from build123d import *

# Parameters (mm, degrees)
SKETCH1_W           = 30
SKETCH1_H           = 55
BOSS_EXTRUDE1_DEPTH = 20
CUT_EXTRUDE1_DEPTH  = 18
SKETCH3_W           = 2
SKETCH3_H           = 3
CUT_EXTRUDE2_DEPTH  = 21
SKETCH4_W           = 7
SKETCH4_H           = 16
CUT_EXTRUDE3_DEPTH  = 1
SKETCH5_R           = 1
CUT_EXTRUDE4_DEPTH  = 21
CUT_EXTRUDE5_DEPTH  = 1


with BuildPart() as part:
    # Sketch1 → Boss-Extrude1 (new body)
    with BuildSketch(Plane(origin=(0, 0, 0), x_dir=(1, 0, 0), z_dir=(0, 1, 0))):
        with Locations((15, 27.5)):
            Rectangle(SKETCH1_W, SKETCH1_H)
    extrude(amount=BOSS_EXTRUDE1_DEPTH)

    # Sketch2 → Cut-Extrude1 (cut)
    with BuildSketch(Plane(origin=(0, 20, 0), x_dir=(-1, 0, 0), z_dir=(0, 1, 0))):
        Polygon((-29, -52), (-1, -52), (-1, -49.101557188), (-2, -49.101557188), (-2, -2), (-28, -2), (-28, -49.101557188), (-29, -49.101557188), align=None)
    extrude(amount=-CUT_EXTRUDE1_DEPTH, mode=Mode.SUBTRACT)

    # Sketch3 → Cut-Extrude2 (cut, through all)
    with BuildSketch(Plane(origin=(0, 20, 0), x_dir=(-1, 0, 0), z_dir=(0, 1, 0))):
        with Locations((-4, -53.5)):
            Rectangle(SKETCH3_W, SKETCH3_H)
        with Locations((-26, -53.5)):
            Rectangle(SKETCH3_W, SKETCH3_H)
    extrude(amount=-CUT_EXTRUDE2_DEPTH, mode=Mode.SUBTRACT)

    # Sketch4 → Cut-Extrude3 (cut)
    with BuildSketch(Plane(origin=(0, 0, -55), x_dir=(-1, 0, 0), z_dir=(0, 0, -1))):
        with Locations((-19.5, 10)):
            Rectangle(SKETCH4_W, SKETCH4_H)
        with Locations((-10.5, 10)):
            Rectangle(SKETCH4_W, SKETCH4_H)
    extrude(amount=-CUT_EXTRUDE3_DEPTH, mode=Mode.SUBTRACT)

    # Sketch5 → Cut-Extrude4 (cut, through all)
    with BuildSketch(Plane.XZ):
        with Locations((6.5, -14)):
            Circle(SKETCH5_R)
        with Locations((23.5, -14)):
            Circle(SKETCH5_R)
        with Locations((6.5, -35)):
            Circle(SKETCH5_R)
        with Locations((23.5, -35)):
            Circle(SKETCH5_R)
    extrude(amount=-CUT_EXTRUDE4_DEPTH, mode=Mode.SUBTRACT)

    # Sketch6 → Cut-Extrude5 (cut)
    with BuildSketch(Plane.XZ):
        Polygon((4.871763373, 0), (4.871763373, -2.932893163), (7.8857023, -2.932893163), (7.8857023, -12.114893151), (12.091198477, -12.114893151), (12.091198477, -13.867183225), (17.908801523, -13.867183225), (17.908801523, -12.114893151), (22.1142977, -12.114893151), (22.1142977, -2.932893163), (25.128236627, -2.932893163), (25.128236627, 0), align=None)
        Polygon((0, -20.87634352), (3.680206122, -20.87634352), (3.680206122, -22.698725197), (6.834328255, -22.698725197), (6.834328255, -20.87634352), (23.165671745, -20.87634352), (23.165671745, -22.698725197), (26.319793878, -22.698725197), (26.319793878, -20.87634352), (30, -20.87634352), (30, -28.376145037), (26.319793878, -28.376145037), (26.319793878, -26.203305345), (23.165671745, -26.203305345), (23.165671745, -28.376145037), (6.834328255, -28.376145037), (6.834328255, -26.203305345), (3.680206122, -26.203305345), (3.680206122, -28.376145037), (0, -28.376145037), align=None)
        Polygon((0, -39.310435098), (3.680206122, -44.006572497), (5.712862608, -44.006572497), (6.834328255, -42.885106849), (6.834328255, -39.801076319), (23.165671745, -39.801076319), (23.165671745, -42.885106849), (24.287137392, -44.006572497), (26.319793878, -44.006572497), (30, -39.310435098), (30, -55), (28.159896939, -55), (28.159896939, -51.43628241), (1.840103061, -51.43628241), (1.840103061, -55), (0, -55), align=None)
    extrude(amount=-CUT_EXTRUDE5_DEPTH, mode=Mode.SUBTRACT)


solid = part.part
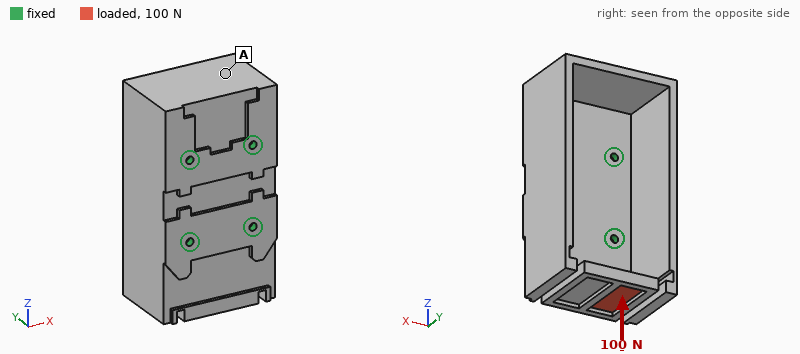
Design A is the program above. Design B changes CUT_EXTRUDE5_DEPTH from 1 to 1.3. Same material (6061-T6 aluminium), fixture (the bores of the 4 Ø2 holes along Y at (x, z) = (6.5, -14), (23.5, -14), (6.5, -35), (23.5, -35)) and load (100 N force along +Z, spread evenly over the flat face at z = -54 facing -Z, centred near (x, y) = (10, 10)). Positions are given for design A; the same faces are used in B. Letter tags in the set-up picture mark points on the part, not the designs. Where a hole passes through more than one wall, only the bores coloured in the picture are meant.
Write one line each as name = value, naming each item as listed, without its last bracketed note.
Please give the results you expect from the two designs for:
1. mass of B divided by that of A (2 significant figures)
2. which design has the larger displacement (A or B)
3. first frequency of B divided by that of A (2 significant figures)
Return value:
mass of B divided by that of A = 0.97
which design has the larger displacement = B
first frequency of B divided by that of A = 0.75
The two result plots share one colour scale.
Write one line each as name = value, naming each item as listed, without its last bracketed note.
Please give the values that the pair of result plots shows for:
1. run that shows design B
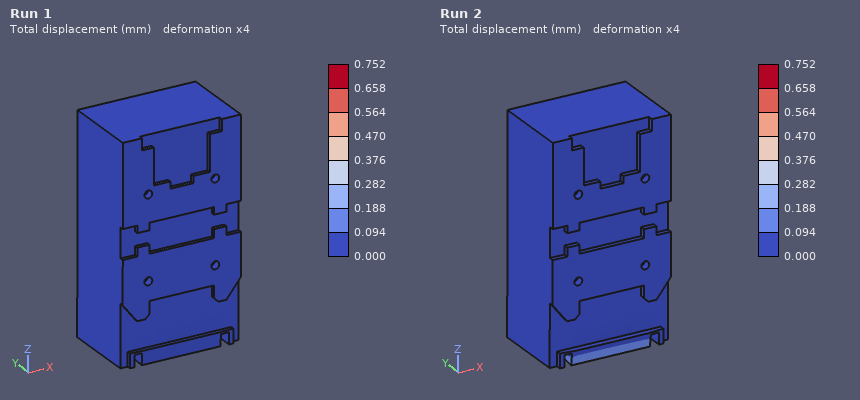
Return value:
run that shows design B = Run 2
